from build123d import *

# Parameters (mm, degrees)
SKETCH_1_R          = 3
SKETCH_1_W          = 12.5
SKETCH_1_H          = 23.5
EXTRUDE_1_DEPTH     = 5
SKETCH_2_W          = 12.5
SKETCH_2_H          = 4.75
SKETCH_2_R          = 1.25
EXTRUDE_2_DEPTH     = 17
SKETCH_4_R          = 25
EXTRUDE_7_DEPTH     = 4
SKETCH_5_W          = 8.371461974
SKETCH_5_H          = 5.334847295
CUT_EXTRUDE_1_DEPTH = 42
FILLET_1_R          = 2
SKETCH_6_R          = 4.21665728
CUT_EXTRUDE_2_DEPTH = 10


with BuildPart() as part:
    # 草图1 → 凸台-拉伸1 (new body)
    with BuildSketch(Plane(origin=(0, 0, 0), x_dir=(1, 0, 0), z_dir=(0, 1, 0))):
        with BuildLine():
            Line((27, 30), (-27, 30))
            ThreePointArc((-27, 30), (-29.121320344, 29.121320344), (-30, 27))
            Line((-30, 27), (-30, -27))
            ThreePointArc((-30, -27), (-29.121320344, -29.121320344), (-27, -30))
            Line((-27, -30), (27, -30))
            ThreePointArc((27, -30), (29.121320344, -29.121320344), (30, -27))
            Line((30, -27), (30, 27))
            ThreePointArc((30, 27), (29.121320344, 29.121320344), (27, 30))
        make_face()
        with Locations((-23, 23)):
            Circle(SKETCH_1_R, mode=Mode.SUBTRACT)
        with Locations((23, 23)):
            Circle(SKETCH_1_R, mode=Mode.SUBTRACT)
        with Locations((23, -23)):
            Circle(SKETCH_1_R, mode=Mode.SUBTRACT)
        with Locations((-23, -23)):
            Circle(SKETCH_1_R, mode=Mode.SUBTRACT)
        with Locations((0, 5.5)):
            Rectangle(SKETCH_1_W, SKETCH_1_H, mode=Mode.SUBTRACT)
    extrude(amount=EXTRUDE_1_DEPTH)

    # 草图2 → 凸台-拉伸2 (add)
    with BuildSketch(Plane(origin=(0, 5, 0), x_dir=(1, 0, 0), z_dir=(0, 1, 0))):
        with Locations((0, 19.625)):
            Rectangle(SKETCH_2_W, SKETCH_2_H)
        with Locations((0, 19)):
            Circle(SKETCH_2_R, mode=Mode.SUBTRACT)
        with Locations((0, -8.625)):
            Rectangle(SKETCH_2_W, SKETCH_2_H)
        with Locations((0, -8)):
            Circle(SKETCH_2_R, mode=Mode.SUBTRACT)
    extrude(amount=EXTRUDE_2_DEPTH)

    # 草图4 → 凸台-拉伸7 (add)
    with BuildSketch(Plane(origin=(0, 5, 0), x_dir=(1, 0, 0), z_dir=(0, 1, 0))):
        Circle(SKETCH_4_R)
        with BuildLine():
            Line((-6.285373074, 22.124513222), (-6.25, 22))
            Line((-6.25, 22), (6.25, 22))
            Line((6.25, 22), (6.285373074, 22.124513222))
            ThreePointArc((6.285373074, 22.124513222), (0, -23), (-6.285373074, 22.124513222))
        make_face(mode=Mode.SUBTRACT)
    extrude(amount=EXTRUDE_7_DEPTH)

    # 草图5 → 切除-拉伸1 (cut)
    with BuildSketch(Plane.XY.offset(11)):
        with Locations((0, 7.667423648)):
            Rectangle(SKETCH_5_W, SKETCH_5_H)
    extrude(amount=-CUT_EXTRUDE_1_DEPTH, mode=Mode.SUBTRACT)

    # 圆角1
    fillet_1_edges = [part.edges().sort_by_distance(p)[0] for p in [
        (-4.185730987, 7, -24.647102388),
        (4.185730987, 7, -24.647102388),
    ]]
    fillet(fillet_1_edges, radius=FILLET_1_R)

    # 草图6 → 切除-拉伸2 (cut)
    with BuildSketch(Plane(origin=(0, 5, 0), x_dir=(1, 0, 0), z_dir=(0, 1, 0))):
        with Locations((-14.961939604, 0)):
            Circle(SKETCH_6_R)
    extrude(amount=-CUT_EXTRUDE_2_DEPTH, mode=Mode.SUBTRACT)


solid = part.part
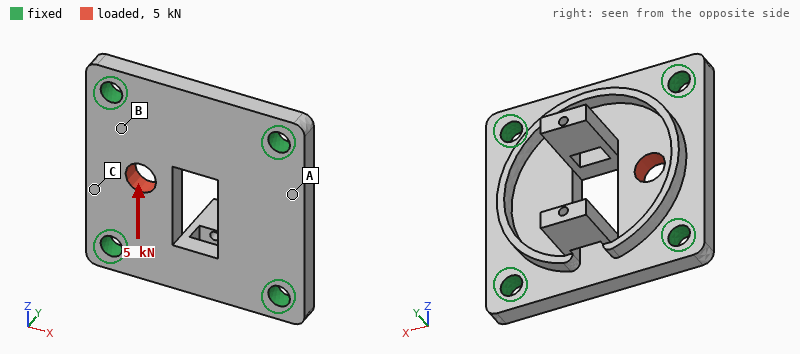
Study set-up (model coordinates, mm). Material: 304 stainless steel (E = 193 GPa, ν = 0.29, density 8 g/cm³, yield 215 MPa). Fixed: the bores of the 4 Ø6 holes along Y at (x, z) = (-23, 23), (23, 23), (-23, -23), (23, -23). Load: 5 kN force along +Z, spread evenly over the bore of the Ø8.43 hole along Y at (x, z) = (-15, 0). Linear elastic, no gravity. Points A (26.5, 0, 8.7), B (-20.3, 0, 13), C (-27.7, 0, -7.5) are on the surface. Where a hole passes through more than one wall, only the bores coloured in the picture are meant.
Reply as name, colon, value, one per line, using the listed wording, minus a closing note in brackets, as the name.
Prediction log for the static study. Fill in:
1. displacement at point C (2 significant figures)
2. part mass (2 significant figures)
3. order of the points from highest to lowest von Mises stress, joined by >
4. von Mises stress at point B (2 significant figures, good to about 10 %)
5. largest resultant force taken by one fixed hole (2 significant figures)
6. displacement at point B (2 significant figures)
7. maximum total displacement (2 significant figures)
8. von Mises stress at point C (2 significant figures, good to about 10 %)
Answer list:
displacement at point C: 1.2 µm
part mass: 150 g
order of the points from highest to lowest von Mises stress, joined by >: B > C > A
von Mises stress at point B: 34 MPa
largest resultant force taken by one fixed hole: 2.3 kN
displacement at point B: 1.4 µm
maximum total displacement: 4.3 µm
von Mises stress at point C: 12 MPa
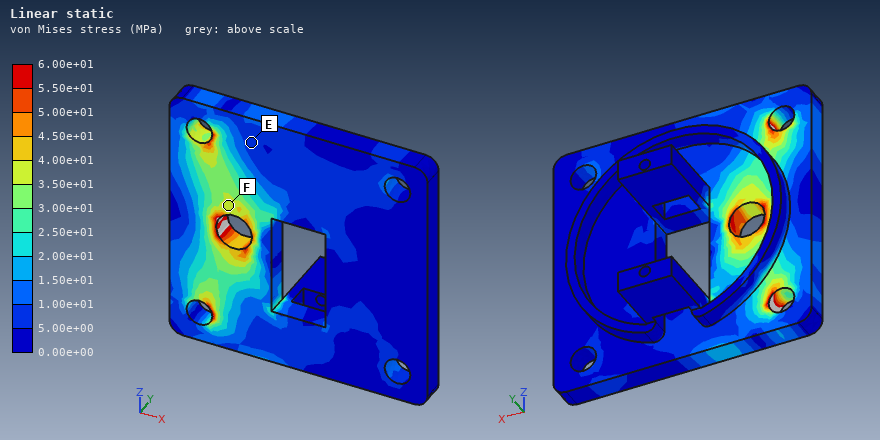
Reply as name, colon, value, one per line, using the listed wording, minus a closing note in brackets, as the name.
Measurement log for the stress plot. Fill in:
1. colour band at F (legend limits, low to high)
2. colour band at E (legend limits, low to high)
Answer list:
colour band at F: 3.50e+01 to 4.00e+01 MPa
colour band at E: 5.00e+00 to 1.00e+01 MPa
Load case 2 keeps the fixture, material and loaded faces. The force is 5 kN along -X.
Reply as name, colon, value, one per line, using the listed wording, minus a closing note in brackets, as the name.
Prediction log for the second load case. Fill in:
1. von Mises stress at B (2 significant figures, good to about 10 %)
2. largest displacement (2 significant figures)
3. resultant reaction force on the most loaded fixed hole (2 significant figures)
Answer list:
von Mises stress at B: 36 MPa
largest displacement: 9.1 µm
resultant reaction force on the most loaded fixed hole: 2.0 kN
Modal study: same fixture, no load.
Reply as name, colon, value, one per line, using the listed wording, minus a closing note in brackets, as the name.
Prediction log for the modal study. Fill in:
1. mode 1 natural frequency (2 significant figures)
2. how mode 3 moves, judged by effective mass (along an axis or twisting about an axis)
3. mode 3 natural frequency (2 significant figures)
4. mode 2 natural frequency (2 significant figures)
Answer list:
mode 1 natural frequency: 6200 Hz
how mode 3 moves, judged by effective mass: along Y
mode 3 natural frequency: 9200 Hz
mode 2 natural frequency: 7400 Hz
